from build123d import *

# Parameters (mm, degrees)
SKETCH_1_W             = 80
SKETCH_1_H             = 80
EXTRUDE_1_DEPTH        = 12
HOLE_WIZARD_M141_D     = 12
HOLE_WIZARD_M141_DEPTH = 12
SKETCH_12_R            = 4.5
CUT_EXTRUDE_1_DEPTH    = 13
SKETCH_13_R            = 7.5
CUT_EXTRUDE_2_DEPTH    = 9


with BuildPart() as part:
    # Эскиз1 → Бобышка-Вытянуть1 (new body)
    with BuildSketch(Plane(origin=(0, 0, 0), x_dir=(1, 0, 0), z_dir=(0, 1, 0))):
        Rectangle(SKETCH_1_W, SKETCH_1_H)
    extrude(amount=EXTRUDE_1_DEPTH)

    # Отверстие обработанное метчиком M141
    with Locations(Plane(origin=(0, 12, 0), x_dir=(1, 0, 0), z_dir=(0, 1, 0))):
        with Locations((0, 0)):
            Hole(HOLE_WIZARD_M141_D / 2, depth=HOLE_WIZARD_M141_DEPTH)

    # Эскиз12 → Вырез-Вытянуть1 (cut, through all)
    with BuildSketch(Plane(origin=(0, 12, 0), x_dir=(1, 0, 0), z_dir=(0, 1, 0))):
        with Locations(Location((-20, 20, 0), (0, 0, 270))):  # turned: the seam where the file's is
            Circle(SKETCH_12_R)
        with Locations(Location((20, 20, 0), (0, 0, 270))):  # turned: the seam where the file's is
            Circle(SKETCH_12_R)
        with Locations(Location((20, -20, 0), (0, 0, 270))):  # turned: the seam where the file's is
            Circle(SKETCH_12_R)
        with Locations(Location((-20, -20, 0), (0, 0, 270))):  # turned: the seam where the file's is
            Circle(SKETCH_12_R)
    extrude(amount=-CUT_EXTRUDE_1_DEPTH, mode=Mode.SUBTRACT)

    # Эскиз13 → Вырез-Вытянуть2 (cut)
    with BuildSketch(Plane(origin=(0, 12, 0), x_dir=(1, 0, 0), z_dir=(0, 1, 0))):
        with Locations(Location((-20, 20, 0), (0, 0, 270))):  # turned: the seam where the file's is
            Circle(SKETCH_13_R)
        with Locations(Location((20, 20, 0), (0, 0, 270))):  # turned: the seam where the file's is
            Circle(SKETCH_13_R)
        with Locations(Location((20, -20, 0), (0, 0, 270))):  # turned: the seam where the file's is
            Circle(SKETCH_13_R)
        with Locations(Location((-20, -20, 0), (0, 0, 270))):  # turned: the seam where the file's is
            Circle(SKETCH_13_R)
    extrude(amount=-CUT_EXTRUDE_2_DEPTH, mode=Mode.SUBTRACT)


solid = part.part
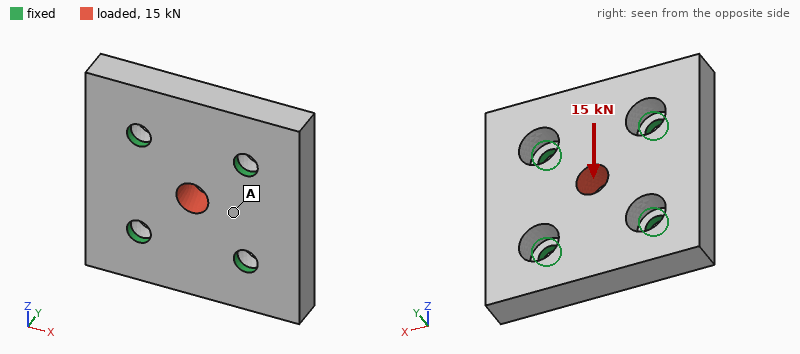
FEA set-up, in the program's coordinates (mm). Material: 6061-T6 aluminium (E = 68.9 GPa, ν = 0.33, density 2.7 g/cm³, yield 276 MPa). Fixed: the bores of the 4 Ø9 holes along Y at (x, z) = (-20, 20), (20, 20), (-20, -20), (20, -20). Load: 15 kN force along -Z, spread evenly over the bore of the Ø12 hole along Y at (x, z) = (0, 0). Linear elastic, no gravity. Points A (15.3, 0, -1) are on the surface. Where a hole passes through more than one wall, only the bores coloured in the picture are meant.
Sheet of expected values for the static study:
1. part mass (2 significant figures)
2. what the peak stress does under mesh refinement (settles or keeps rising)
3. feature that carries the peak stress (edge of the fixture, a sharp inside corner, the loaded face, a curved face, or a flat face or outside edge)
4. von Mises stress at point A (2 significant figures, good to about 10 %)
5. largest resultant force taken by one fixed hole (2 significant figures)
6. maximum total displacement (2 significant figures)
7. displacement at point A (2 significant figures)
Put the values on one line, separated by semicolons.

180 g; keeps rising; edge of the fixture; 17 MPa; 3.9 kN; 16 µm; 6.7 µm
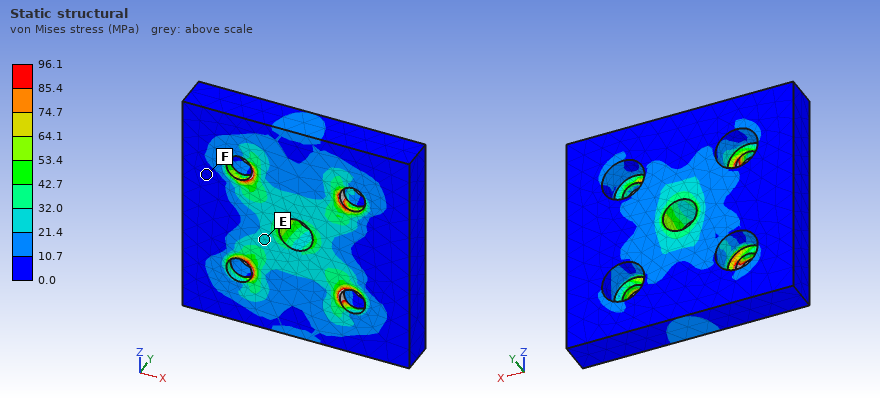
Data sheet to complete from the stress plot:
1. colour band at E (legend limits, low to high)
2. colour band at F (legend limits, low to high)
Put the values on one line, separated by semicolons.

21.4 to 32.0 MPa; 0.0 to 10.7 MPa
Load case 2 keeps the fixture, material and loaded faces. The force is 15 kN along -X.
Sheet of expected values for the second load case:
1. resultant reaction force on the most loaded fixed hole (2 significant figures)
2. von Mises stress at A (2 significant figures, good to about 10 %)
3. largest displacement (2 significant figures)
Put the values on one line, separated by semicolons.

3.9 kN; 22 MPa; 16 µm
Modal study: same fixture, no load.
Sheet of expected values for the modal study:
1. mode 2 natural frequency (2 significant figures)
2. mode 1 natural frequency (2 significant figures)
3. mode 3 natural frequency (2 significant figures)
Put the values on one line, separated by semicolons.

9800 Hz; 9800 Hz; 11 kHz
